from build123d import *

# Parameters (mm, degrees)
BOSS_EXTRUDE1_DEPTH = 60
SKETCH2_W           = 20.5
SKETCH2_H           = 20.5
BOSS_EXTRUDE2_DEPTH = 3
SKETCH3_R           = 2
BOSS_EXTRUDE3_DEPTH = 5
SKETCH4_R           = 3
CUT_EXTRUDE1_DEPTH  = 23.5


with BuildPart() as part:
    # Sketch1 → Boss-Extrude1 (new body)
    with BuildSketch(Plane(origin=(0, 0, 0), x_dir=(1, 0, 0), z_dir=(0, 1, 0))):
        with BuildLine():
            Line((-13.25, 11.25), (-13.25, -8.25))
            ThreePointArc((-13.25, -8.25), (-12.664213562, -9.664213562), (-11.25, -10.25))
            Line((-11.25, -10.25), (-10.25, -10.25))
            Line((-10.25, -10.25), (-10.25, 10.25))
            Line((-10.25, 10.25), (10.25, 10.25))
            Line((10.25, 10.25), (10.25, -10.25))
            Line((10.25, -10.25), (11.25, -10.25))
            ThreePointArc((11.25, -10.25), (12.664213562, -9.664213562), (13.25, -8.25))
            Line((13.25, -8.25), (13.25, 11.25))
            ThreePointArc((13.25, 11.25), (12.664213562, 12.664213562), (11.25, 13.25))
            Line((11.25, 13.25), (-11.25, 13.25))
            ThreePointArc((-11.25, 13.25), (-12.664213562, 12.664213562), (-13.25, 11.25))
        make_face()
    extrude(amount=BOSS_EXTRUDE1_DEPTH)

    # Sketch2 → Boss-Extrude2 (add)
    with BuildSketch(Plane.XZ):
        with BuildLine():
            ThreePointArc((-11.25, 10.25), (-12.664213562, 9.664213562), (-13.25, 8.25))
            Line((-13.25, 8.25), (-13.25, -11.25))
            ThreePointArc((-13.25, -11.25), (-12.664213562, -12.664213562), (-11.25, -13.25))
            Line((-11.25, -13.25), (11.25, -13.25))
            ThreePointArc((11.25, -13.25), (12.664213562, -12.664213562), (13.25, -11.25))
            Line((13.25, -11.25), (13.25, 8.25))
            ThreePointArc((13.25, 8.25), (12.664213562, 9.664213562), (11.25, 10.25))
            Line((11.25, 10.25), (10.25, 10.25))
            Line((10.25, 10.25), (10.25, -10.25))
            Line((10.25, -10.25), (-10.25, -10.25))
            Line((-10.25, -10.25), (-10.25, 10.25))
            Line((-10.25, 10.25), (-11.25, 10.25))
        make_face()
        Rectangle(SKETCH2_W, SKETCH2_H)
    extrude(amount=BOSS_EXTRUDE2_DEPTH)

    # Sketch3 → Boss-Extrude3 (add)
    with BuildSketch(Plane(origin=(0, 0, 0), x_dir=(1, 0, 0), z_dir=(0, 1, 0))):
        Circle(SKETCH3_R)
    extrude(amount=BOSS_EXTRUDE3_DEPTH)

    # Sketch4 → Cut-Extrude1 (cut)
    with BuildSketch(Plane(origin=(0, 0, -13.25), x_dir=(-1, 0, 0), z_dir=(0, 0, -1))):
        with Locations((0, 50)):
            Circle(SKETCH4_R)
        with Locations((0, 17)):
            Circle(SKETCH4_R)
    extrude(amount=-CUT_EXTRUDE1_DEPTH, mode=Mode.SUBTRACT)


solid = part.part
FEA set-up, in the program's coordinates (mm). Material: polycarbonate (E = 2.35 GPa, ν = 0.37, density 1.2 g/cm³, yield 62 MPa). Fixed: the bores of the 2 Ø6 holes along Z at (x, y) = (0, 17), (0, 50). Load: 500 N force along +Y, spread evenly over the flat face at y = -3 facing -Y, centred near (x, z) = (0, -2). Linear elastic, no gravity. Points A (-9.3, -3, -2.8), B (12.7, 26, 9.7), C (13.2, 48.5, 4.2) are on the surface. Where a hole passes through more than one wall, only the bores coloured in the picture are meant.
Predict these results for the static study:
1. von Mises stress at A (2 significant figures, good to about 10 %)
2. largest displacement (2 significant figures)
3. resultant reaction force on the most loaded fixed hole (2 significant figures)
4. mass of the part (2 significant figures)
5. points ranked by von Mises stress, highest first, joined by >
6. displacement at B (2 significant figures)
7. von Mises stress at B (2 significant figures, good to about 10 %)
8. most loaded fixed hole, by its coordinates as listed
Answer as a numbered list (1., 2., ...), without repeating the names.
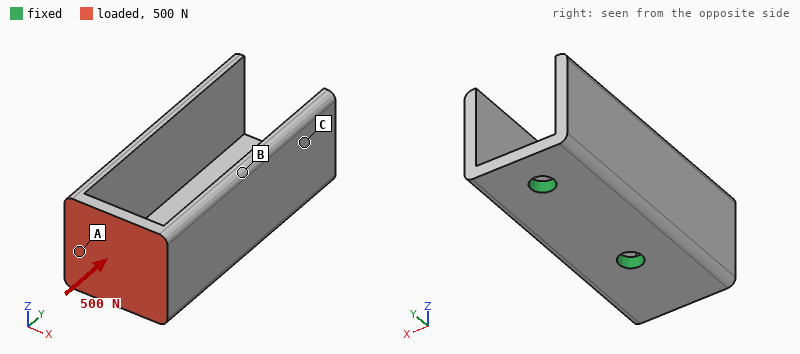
1. 7.4 MPa
2. 0.60 mm
3. 340 N
4. 16 g
5. A > B > C
6. 0.26 mm
7. 4.5 MPa
8. (0, 17)
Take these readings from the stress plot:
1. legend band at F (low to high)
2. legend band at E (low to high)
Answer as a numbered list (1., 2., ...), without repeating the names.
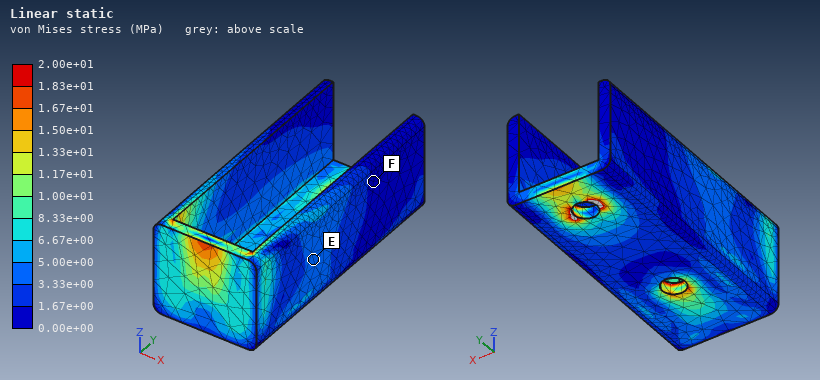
1. 0.00e+00 to 1.67e+00 MPa
2. 3.33e+00 to 5.00e+00 MPa
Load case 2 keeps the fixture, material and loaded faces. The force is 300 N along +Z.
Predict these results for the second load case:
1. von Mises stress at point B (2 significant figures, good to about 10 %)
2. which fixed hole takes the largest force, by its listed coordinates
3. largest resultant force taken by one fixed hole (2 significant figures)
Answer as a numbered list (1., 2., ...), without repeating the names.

1. 7.2 MPa
2. (0, 17)
3. 450 N
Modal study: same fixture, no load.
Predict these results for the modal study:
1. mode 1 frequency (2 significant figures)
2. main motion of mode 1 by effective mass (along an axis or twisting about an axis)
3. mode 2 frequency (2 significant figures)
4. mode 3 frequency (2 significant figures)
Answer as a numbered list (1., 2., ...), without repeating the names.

1. 790 Hz
2. along X
3. 1000 Hz
4. 1200 Hz
